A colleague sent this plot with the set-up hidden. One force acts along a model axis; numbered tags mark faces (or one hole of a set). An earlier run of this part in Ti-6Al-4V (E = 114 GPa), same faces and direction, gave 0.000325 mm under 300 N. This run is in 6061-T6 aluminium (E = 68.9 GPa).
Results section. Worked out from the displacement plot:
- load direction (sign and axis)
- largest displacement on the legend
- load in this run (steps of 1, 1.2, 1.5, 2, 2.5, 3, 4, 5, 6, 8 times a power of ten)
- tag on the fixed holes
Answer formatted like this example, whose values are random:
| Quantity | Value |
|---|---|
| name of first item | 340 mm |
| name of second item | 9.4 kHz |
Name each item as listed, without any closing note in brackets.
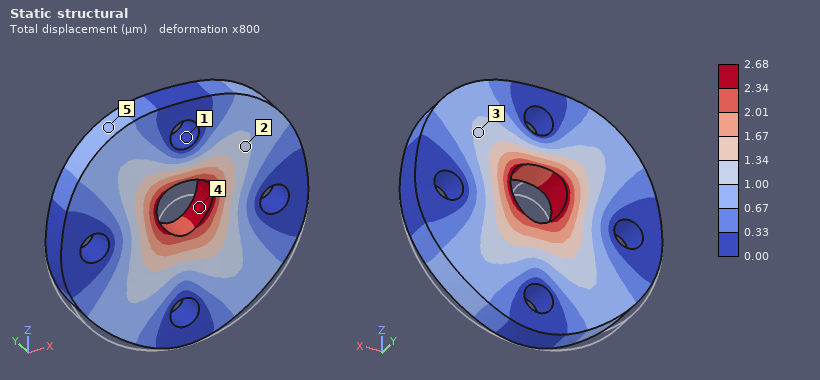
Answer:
| Quantity | Value |
|---|---|
| load direction | +Z |
| largest displacement on the legend | 2.68 µm |
| load in this run | 1.5 kN |
| tag on the fixed holes | 1 |
